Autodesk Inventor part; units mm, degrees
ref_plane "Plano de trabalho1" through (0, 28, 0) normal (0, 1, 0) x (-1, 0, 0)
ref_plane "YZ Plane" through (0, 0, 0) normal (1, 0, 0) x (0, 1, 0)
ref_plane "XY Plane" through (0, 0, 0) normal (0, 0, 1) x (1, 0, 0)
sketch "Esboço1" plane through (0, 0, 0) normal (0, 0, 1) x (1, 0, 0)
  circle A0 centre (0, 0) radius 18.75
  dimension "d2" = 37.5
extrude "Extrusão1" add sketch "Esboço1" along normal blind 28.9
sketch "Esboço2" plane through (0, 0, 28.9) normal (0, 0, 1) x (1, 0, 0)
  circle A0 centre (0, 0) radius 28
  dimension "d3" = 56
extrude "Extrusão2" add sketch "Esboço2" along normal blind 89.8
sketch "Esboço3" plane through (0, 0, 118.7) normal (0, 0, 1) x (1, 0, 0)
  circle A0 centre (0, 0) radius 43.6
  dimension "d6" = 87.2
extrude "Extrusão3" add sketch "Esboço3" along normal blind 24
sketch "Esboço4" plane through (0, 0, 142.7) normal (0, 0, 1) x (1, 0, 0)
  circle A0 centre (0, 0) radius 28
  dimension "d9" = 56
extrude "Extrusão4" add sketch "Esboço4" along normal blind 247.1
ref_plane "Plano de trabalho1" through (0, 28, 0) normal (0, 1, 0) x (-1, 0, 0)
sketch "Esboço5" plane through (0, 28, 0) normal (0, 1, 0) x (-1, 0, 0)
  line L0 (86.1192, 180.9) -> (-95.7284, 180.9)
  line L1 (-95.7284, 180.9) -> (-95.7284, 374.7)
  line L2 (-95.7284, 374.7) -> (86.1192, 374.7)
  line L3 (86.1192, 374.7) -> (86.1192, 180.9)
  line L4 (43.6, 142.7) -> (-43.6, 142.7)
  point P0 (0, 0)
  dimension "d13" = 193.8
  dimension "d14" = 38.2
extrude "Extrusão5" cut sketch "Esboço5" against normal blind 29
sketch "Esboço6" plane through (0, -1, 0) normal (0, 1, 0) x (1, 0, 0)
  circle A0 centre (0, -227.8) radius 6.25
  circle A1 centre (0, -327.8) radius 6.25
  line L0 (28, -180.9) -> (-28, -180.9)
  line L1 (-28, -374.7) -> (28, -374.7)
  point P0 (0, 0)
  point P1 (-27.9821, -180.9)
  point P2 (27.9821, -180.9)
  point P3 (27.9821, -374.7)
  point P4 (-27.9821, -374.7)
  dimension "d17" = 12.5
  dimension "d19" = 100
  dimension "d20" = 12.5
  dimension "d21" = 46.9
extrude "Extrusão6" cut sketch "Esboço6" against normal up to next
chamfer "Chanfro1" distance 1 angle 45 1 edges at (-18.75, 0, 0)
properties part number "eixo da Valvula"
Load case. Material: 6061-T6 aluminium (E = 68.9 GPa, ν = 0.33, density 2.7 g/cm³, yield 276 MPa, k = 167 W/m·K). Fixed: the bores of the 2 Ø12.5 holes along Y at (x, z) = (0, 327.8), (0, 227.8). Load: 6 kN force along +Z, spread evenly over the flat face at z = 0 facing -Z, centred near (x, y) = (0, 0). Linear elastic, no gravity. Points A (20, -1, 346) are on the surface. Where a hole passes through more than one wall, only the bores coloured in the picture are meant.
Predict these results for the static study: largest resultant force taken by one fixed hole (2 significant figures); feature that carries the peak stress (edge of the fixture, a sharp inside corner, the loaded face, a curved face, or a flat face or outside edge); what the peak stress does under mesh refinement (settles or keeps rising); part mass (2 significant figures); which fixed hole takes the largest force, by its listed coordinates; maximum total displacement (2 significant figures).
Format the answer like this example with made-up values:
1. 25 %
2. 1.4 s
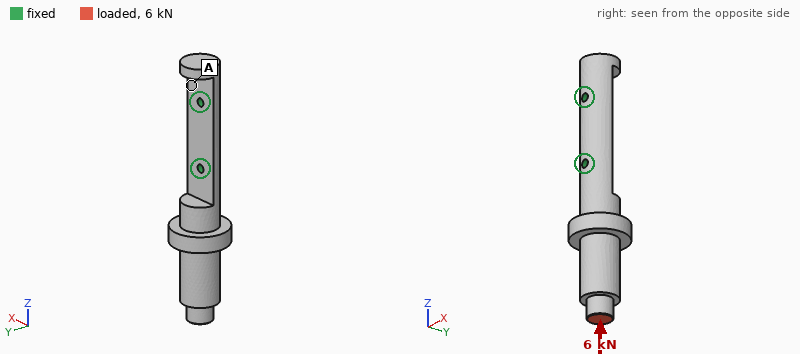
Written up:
1. 5.4 kN
2. edge of the fixture
3. keeps rising
4. 2.0 kg
5. (0, 227.8)
6. 0.21 mm
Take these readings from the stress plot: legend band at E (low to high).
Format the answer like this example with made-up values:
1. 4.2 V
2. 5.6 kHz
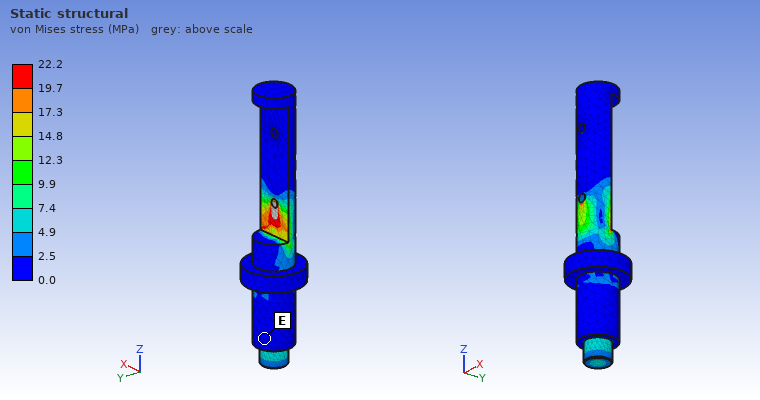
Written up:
1. 0.0 to 2.5 MPa
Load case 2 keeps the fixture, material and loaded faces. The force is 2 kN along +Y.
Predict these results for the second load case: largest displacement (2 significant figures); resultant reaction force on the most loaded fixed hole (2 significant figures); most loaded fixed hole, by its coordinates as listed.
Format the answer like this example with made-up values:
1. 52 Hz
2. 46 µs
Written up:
1. 1.2 mm
2. 2.8 kN
3. (0, 227.8)
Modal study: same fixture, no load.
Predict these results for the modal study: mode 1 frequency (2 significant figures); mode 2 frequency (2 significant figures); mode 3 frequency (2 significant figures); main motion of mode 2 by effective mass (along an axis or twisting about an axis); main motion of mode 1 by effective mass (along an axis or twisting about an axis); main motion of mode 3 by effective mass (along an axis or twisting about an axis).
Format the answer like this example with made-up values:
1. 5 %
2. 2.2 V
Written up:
1. 330 Hz
2. 500 Hz
3. 1600 Hz
4. along X
5. along Y
6. twisting about Z
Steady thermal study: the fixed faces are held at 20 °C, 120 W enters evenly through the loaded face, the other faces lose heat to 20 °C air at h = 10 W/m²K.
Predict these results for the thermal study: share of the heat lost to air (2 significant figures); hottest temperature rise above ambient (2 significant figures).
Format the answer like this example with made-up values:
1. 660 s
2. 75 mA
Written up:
1. 17 %
2. 86 K
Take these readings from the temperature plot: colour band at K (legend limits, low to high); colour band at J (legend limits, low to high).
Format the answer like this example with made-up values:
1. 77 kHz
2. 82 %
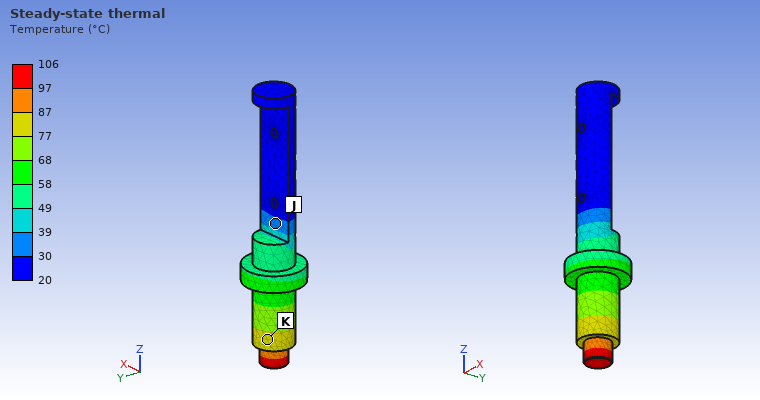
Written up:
1. 77 to 87 °C
2. 30 to 39 °C
